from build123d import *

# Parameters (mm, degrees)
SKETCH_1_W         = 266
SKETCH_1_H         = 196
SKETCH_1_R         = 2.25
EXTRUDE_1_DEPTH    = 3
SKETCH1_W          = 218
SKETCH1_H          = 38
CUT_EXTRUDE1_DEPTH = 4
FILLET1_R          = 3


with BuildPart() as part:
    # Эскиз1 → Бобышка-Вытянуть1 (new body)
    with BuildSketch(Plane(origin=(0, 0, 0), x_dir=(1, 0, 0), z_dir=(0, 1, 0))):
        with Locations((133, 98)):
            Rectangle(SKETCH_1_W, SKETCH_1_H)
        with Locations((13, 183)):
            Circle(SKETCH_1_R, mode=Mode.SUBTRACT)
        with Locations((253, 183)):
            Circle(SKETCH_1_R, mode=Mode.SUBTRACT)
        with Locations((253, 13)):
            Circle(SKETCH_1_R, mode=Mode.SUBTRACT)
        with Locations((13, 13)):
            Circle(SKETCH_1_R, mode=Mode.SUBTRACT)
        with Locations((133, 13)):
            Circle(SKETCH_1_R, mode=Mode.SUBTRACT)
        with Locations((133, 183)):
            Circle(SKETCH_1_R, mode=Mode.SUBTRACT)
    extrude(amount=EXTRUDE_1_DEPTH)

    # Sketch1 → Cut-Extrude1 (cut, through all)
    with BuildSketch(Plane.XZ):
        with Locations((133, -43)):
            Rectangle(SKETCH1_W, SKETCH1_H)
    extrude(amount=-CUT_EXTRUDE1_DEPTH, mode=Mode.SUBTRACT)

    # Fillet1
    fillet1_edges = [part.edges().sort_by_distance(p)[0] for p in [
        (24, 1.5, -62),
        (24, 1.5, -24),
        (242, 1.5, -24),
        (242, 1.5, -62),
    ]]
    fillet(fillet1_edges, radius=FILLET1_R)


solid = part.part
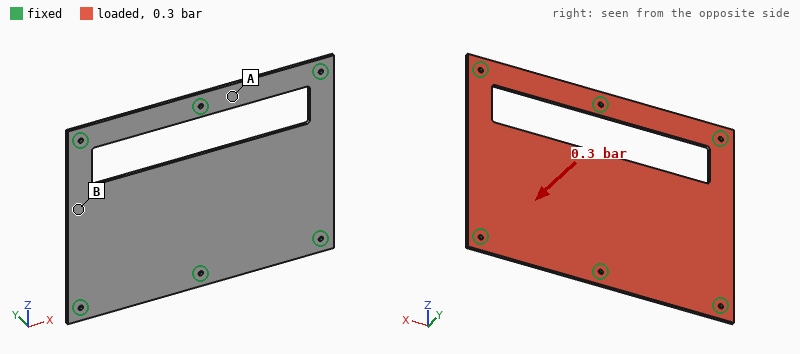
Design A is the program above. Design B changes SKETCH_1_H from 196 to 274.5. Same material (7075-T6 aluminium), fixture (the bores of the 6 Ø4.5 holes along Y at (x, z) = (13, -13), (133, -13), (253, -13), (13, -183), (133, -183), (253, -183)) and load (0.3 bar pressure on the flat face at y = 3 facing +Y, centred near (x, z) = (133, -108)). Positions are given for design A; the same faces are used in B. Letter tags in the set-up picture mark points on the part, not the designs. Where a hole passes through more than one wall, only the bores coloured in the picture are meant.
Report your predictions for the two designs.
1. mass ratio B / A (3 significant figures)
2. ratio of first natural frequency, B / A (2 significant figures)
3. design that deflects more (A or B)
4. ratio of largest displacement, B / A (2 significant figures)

1.48
1.0
A
0.91
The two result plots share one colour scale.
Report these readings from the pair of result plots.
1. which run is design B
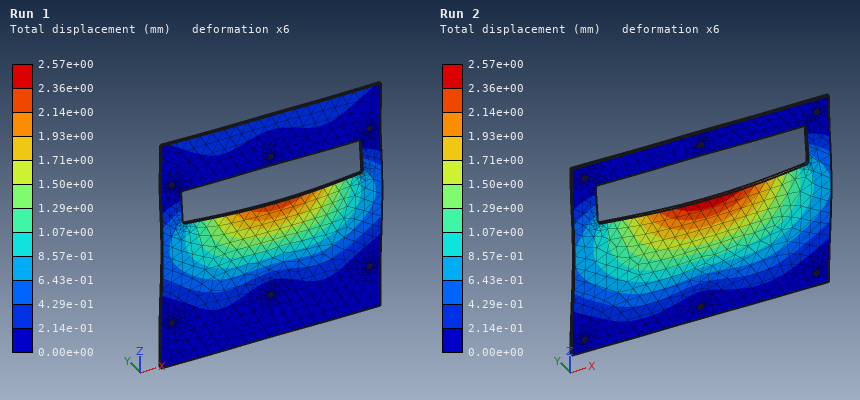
Run 1
